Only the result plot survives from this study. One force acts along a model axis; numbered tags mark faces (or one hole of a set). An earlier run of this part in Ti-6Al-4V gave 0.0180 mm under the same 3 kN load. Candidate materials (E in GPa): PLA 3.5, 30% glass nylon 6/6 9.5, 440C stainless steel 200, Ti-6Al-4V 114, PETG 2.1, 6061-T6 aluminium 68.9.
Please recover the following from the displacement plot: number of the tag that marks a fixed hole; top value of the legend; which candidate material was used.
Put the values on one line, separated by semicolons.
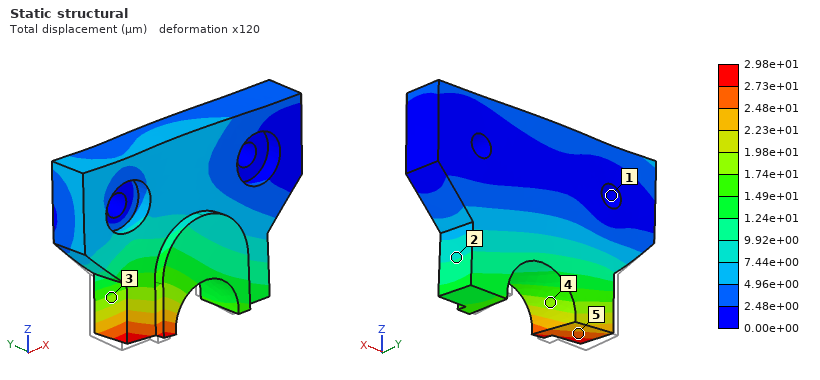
1; 2.98e+01 µm; 6061-T6 aluminium
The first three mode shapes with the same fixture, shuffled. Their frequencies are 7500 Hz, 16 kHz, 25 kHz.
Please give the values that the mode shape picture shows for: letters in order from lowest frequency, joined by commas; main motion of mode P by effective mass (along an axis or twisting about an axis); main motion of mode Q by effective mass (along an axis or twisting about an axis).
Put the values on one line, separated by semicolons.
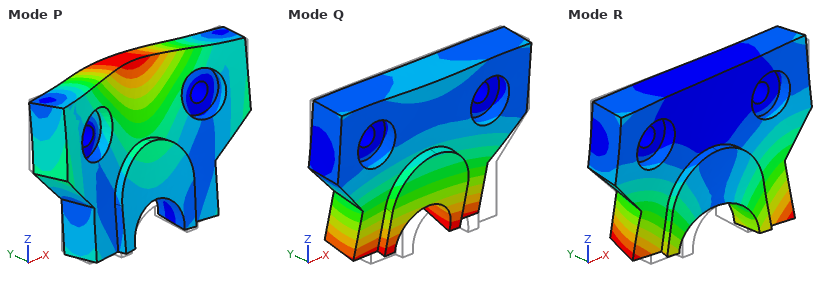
Q, R, P; along Y; along Y
